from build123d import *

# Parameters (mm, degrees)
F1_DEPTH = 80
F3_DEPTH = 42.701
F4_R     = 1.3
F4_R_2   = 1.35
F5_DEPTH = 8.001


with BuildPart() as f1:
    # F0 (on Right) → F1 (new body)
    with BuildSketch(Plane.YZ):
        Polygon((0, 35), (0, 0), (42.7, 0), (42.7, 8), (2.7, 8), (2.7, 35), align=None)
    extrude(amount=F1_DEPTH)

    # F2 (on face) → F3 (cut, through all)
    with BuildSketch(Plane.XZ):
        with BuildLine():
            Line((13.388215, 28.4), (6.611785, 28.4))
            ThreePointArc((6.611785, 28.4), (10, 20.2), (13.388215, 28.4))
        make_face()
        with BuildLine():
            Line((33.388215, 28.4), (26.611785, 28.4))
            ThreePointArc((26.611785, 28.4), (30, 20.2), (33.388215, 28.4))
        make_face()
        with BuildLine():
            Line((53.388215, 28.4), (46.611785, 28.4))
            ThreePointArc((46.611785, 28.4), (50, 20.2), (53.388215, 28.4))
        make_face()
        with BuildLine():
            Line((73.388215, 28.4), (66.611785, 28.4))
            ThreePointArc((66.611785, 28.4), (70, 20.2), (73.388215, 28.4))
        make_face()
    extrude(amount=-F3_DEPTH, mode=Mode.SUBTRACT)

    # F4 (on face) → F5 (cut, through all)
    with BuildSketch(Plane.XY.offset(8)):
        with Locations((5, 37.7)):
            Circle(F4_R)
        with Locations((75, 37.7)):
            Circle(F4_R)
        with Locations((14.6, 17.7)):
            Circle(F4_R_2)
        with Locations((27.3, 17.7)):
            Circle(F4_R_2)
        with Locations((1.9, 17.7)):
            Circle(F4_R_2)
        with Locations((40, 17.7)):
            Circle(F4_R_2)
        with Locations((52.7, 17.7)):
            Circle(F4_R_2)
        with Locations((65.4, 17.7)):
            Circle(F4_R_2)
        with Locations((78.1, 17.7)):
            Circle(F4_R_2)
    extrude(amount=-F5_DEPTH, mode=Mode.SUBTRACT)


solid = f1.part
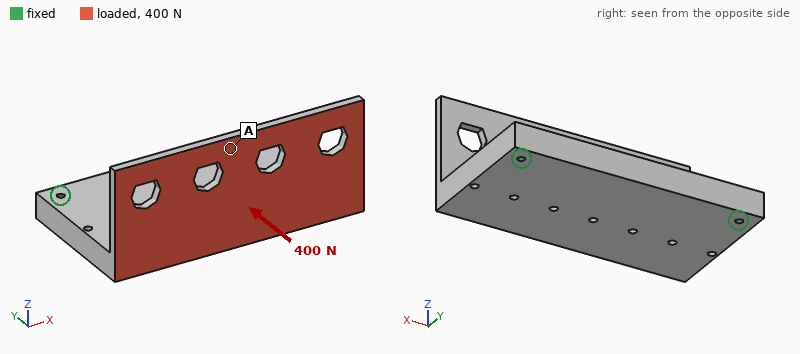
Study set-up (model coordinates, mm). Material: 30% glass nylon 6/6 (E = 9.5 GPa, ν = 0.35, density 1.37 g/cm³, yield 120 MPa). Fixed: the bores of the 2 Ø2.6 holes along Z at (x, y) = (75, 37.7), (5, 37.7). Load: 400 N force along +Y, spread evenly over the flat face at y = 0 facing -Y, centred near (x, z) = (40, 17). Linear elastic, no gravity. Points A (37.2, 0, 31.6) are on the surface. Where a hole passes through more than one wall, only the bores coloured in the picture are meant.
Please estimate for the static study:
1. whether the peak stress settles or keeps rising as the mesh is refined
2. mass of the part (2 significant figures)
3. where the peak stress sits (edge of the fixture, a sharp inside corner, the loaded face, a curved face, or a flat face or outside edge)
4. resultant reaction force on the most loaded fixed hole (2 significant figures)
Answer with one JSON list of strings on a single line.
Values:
["keeps rising", "44 g", "edge of the fixture", "220 N"]
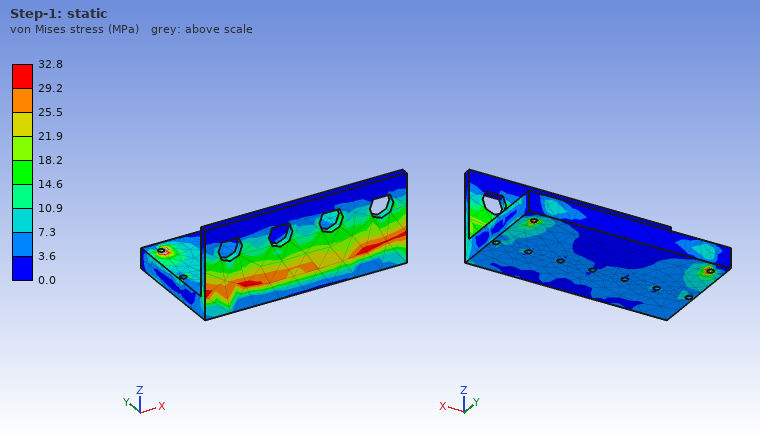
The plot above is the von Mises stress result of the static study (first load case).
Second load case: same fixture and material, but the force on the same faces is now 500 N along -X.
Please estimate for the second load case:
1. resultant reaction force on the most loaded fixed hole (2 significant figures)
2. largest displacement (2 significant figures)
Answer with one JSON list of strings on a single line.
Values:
["380 N", "0.17 mm"]
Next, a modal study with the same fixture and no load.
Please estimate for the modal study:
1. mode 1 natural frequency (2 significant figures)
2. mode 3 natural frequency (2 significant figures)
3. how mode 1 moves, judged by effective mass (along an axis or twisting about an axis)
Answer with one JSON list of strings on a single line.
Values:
["950 Hz", "1700 Hz", "along Z"]
